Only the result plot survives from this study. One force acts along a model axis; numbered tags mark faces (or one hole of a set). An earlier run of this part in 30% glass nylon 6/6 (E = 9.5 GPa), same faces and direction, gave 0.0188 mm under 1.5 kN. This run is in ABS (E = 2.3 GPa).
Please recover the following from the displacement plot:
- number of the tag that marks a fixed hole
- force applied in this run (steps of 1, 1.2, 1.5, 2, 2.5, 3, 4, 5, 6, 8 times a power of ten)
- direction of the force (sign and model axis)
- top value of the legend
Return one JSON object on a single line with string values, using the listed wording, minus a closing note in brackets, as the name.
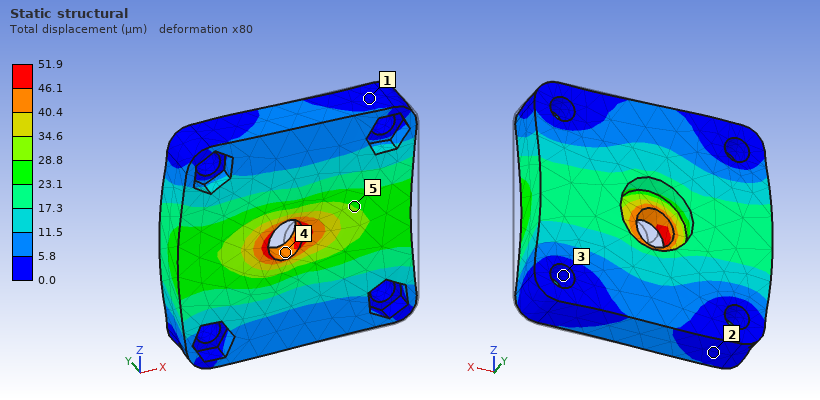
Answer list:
{"number of the tag that marks a fixed hole": "3", "force applied in this run": "1 kN", "direction of the force": "-X", "top value of the legend": "51.9 µm"}
